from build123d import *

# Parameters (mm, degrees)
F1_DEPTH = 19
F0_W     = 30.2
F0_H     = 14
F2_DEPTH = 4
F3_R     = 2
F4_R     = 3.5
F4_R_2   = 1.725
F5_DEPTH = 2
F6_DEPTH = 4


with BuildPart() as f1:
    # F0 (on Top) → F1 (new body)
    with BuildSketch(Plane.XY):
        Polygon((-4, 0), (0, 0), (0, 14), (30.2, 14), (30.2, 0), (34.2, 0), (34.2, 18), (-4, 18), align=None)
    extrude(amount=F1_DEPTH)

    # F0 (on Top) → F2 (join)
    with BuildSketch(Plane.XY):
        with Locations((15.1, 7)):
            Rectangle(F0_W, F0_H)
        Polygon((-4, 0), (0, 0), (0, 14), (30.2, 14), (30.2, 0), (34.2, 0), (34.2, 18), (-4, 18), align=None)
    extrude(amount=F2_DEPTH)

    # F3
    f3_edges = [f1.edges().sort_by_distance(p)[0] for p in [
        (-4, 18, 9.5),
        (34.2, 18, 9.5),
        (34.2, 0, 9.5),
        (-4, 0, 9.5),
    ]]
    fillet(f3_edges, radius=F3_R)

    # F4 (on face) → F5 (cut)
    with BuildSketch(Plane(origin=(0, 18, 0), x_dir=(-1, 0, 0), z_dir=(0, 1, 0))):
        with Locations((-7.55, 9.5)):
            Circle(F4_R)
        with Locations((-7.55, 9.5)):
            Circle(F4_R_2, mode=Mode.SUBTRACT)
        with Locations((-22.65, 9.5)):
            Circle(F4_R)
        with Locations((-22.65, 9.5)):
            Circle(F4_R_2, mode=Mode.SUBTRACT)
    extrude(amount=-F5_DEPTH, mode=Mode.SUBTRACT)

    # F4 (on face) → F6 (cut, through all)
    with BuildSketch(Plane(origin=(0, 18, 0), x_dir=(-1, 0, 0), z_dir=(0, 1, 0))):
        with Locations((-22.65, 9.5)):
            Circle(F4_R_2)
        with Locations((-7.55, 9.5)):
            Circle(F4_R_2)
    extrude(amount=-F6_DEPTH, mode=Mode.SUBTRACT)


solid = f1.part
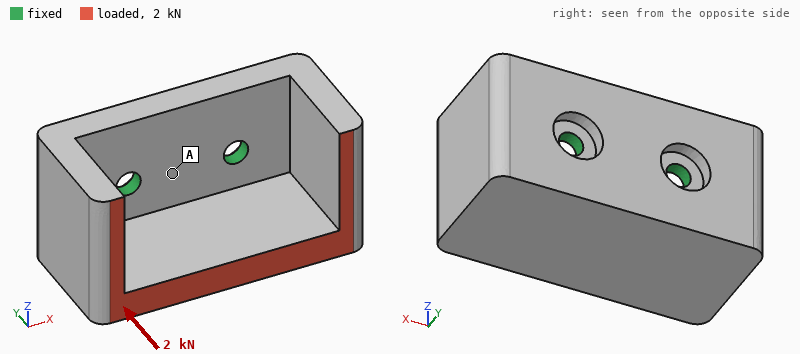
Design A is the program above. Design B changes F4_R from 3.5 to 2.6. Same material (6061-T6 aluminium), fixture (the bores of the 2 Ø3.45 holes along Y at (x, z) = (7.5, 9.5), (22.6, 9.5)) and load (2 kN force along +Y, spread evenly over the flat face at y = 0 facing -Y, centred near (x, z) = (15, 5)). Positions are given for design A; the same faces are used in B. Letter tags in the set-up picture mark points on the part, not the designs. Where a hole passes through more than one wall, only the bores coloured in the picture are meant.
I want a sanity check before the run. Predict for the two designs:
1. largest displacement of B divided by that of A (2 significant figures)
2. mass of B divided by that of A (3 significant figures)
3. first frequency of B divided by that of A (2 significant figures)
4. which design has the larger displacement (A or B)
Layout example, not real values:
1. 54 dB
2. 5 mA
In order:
1. 0.87
2. 1.01
3. 1.1
4. A
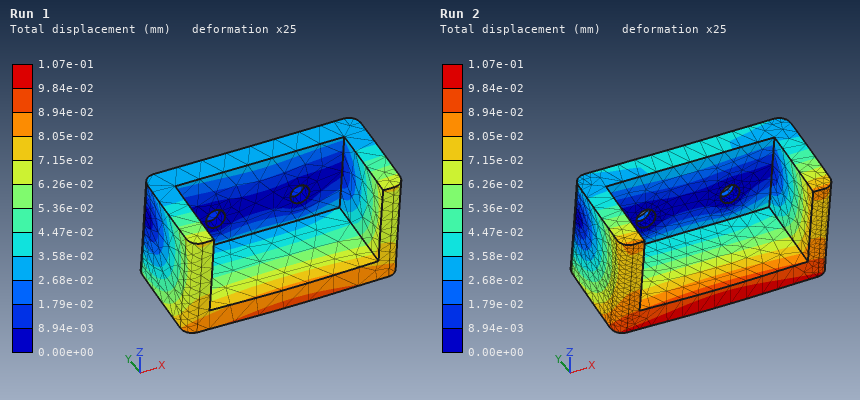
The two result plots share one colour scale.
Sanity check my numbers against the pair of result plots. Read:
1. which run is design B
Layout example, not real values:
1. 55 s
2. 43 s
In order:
1. Run 1
